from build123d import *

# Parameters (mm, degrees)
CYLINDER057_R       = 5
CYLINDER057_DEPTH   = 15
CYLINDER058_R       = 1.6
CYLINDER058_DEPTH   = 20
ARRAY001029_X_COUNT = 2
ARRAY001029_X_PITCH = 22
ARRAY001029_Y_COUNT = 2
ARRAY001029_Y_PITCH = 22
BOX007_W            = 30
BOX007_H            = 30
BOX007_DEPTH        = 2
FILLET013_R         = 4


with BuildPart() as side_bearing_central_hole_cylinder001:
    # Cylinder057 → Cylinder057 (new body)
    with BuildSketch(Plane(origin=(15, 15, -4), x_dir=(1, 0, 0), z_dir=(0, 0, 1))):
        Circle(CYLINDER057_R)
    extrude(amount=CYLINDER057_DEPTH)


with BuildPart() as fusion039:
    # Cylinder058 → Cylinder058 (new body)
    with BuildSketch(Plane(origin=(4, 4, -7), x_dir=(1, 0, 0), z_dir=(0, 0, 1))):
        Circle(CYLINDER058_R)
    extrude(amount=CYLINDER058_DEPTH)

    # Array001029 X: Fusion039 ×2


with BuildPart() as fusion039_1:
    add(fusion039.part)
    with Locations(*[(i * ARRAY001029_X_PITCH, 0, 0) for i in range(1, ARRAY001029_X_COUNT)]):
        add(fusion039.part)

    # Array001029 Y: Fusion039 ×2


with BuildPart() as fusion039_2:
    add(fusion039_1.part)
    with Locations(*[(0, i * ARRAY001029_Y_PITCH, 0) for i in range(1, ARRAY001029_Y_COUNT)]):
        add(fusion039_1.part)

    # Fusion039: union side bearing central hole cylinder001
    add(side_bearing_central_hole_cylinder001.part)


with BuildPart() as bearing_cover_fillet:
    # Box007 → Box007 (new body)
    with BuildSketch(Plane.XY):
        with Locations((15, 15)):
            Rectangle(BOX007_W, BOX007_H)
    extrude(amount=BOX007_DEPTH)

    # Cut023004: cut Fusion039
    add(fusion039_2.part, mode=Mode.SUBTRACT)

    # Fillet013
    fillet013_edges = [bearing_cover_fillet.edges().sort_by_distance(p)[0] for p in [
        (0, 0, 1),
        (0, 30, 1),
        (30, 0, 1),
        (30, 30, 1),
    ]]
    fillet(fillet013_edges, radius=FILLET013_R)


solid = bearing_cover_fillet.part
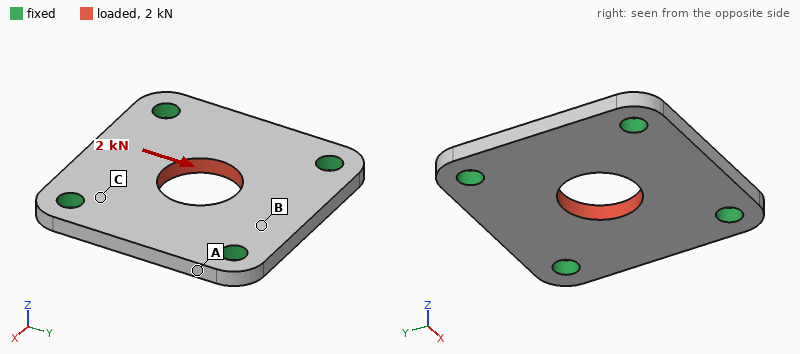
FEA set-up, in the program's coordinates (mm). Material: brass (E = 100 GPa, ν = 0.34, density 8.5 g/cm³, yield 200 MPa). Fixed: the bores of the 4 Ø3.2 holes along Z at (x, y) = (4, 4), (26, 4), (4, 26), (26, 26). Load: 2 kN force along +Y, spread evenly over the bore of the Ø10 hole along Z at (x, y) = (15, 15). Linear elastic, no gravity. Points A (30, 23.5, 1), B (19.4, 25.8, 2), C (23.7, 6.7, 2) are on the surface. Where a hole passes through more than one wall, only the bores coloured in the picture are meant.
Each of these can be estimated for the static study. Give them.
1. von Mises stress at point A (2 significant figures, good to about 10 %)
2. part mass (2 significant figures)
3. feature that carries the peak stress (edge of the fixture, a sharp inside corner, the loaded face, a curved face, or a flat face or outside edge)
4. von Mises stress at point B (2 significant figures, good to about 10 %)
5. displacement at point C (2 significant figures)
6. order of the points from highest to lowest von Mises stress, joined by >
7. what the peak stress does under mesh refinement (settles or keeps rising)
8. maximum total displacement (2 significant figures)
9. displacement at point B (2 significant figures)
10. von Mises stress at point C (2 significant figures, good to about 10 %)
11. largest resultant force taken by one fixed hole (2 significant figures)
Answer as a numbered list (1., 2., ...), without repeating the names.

1. 6.7 MPa
2. 13 g
3. edge of the fixture
4. 22 MPa
5. 1.2 µm
6. C > B > A
7. keeps rising
8. 5.5 µm
9. 3.3 µm
10. 43 MPa
11. 540 N
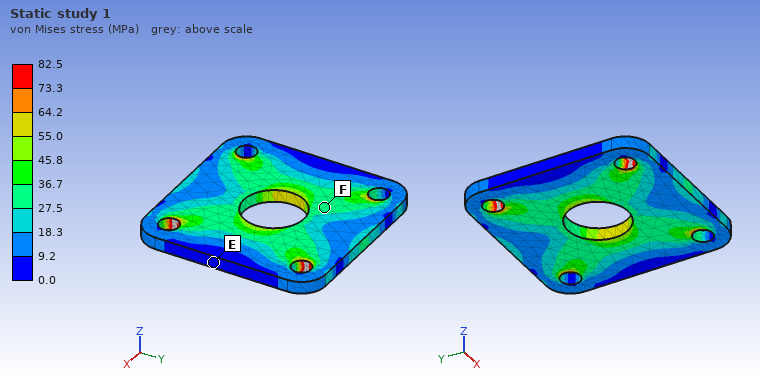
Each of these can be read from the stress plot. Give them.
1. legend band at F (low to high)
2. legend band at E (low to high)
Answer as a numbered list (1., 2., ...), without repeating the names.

1. 27.5 to 36.7 MPa
2. 0.0 to 9.2 MPa
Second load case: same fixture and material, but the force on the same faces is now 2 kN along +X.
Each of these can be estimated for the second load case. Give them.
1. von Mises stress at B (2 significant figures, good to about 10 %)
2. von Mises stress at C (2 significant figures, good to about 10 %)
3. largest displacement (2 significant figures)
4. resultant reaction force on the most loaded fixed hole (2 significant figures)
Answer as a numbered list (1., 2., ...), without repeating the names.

1. 19 MPa
2. 43 MPa
3. 5.5 µm
4. 540 N
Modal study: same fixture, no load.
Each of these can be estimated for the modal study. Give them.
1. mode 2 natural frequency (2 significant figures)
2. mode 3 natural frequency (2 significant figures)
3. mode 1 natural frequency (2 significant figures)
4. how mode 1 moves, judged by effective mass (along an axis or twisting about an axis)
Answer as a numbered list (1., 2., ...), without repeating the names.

1. 17 kHz
2. 17 kHz
3. 13 kHz
4. along Z
